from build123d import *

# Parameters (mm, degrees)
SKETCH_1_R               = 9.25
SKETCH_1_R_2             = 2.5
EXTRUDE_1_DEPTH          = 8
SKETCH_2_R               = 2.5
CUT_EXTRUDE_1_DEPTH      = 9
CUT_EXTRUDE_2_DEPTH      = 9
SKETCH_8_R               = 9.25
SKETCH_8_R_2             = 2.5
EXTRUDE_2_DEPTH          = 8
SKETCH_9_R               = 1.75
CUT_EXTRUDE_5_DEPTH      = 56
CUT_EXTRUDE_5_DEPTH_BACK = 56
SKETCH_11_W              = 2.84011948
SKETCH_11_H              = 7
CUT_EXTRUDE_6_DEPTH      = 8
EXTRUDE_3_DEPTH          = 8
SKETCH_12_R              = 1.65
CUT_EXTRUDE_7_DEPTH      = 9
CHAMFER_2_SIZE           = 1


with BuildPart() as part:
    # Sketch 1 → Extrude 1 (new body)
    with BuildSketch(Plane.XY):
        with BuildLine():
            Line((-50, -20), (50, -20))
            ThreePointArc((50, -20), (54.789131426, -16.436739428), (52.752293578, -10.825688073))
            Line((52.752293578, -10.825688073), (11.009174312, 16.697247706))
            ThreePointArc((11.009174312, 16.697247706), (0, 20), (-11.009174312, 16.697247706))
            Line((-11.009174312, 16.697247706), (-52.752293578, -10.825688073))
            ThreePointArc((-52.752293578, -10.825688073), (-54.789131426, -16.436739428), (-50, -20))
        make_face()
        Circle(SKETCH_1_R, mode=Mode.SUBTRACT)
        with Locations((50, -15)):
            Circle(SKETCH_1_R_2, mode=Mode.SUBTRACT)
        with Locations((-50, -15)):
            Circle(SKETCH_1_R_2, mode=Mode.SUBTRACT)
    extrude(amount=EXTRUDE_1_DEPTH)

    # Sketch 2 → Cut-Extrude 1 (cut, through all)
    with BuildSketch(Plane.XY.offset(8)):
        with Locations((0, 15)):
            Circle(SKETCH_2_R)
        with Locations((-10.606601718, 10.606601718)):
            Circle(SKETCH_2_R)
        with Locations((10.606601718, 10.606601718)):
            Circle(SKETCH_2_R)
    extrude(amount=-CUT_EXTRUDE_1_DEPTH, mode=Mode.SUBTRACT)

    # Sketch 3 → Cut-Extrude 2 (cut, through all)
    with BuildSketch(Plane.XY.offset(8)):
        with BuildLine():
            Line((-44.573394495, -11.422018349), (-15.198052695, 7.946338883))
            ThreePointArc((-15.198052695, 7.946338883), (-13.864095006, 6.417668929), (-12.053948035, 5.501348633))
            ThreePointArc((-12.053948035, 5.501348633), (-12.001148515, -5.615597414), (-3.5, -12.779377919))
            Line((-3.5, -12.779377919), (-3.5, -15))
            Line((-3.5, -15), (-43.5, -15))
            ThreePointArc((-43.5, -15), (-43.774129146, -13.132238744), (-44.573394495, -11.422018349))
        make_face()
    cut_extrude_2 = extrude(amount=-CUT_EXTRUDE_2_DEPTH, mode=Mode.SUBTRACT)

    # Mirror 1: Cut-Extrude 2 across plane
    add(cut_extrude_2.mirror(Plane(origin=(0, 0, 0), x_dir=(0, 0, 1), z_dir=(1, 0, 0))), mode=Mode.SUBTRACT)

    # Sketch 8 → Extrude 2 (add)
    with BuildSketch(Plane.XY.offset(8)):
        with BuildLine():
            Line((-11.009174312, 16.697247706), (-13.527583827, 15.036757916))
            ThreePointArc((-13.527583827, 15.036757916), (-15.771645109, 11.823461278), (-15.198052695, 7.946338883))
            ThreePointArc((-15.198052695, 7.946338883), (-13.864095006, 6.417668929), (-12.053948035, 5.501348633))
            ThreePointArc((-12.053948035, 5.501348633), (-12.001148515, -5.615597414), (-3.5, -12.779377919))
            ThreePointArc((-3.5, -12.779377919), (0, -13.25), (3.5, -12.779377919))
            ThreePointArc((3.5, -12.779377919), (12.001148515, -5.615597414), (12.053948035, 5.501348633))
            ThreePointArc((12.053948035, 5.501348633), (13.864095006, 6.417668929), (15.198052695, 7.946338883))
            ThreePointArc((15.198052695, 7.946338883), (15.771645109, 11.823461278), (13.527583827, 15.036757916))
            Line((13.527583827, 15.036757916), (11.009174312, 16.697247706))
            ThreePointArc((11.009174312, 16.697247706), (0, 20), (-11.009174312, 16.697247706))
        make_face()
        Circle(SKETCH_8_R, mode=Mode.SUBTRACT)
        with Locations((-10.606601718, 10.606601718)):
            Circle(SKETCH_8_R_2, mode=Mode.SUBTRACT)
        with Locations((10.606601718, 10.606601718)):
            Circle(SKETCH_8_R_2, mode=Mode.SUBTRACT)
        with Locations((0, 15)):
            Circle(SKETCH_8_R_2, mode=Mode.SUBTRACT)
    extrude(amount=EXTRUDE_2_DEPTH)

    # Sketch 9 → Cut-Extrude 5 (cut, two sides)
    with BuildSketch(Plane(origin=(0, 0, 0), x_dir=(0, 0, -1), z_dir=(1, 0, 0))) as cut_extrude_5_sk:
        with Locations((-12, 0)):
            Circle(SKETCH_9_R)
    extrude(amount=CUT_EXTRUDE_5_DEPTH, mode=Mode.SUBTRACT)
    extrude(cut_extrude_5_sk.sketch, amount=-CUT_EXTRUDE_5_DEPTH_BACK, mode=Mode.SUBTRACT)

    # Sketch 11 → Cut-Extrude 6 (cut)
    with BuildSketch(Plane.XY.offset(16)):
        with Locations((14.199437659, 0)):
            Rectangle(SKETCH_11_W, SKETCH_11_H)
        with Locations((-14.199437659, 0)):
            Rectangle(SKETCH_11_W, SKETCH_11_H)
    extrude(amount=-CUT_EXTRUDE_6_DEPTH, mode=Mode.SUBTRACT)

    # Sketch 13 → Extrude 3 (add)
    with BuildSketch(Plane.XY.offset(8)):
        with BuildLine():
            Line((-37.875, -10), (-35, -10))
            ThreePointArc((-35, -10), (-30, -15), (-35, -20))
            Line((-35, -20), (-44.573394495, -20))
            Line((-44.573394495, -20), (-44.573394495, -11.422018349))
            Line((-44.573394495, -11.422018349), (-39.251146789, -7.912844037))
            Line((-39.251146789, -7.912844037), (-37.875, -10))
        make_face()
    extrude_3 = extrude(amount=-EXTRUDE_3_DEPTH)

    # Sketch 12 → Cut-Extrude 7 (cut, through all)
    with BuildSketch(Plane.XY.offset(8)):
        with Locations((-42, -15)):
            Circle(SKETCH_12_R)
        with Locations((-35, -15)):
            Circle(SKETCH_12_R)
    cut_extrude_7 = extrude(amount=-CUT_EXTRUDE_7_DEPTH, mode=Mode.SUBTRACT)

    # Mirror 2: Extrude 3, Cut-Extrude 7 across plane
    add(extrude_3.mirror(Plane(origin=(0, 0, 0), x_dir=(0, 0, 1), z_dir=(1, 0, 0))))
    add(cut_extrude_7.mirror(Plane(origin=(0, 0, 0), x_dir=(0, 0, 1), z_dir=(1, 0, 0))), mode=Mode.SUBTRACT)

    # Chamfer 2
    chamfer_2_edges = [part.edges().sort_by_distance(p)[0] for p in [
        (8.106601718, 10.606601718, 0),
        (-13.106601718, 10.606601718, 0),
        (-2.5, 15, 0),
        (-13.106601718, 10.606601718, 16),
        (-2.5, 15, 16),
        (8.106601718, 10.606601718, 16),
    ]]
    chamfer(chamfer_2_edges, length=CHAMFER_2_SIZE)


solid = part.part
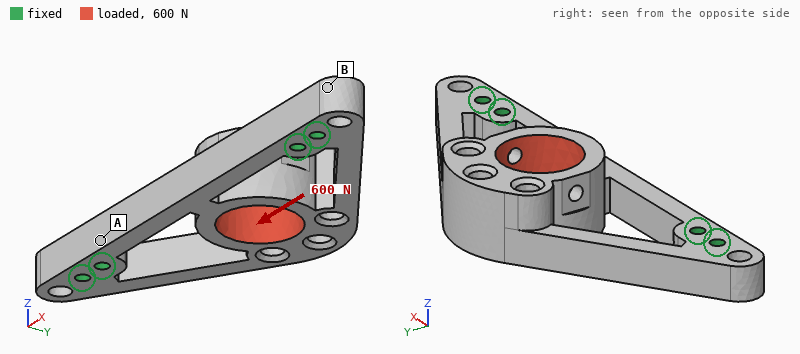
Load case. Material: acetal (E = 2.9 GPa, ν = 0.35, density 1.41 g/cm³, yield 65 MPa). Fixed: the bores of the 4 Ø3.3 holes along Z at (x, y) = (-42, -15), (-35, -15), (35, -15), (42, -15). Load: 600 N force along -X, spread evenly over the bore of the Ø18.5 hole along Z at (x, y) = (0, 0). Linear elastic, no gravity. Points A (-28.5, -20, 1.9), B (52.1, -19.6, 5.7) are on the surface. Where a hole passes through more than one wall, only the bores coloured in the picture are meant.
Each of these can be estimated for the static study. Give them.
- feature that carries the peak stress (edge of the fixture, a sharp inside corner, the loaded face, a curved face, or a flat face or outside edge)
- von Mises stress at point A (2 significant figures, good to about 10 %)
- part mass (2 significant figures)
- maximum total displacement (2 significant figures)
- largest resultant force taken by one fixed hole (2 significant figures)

a flat face or outside edge
6.6 MPa
23 g
0.25 mm
200 N
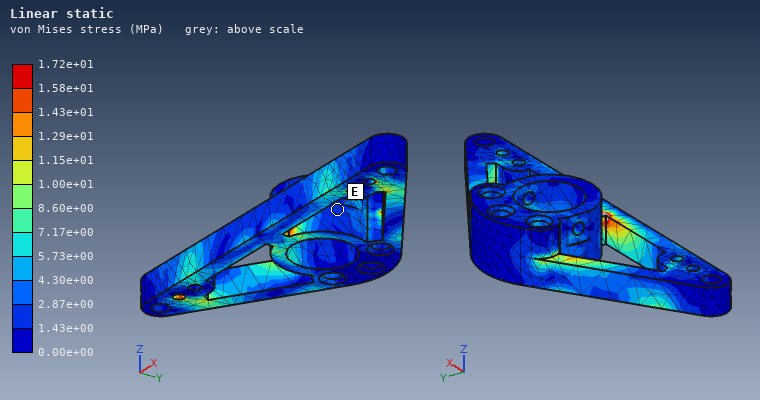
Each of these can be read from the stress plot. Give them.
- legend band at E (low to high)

1.43e+00 to 2.87e+00 MPa
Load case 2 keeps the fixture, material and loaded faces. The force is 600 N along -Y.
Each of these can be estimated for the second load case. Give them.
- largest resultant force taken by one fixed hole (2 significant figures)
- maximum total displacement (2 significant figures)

450 N
1.4 mm
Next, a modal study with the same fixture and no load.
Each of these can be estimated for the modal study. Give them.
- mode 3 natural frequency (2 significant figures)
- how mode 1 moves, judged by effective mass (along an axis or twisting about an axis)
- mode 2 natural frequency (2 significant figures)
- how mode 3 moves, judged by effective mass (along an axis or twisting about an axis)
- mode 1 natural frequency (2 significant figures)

1900 Hz
along Z
1500 Hz
along Y
580 Hz
